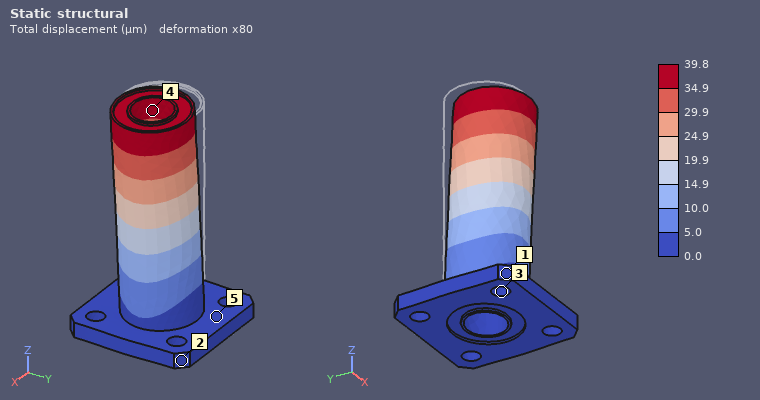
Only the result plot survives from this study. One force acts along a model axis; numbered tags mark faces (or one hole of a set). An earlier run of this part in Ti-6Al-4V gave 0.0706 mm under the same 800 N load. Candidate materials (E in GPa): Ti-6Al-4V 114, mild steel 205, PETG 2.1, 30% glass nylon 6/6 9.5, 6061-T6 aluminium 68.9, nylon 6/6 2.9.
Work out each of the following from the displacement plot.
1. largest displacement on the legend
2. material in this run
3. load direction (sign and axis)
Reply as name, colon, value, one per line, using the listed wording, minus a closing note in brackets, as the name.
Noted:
largest displacement on the legend: 39.8 µm
material in this run: mild steel
load direction: +X
